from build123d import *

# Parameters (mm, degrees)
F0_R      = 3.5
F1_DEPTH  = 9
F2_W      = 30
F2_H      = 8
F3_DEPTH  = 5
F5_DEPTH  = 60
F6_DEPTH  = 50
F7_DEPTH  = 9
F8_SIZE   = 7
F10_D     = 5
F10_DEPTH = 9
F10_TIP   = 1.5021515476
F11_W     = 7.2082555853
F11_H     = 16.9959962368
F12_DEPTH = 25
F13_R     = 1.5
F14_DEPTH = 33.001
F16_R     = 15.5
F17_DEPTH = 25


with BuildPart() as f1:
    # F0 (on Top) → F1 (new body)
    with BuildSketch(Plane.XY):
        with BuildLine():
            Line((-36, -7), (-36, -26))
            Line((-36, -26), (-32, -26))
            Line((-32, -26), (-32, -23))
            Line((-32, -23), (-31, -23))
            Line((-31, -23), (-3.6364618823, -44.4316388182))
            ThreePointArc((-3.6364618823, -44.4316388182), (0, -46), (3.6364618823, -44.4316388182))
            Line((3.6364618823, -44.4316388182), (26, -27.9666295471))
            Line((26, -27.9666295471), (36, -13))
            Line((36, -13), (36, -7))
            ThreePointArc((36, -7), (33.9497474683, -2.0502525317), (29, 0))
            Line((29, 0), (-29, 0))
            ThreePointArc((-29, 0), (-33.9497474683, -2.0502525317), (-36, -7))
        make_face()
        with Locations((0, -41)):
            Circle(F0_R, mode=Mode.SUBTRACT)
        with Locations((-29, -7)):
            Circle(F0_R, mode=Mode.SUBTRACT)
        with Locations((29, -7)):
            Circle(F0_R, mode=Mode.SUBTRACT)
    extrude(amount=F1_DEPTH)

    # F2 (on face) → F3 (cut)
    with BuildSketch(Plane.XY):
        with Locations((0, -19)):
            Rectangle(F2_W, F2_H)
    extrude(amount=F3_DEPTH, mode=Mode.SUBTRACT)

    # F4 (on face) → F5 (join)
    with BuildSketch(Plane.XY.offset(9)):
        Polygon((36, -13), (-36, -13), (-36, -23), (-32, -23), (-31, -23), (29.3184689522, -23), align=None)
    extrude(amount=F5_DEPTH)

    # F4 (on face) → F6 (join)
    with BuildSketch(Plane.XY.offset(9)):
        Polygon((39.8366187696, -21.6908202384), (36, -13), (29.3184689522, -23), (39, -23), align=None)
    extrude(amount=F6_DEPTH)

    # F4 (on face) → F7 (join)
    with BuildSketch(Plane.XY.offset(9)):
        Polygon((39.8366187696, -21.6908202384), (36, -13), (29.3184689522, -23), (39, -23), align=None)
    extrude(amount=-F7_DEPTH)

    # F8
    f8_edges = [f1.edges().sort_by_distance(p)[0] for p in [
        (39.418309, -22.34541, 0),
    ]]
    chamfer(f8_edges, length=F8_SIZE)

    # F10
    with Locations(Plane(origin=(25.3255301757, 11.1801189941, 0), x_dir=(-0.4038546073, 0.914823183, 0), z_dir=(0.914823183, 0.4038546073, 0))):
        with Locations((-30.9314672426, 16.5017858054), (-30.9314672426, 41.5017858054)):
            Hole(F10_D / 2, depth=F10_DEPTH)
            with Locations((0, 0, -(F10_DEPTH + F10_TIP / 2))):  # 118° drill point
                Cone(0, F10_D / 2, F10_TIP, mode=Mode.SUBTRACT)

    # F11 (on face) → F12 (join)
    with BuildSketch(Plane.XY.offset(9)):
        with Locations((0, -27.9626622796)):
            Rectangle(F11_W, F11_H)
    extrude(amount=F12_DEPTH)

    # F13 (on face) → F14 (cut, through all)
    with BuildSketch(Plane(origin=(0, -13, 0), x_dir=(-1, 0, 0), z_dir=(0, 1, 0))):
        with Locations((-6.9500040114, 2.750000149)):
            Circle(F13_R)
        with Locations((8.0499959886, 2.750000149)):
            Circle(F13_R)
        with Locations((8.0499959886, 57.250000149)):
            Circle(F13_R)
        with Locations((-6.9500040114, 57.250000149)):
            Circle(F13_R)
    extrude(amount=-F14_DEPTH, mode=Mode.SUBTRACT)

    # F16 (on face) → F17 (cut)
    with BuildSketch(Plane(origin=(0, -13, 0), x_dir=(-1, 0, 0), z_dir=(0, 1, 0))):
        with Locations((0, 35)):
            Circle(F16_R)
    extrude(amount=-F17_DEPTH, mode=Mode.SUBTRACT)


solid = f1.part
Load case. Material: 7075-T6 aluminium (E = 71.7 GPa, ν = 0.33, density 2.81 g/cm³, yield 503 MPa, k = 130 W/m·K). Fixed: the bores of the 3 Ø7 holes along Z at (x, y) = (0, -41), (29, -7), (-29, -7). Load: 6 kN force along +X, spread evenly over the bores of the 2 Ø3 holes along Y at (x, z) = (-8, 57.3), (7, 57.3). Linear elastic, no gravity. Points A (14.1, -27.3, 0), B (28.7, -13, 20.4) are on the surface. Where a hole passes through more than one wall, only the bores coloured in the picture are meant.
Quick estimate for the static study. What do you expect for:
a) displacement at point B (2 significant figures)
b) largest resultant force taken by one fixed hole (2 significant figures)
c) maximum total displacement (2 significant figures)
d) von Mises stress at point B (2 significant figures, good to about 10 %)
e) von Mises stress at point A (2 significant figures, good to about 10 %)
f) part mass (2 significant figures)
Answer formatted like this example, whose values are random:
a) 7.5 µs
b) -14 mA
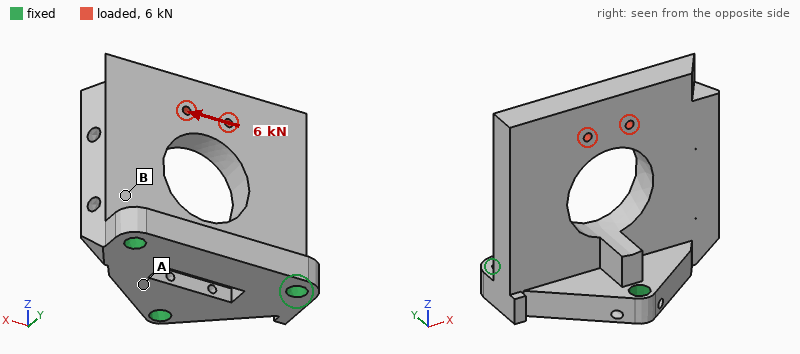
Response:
a) 0.036 mm
b) 5.7 kN
c) 0.13 mm
d) 52 MPa
e) 21 MPa
f) 160 g
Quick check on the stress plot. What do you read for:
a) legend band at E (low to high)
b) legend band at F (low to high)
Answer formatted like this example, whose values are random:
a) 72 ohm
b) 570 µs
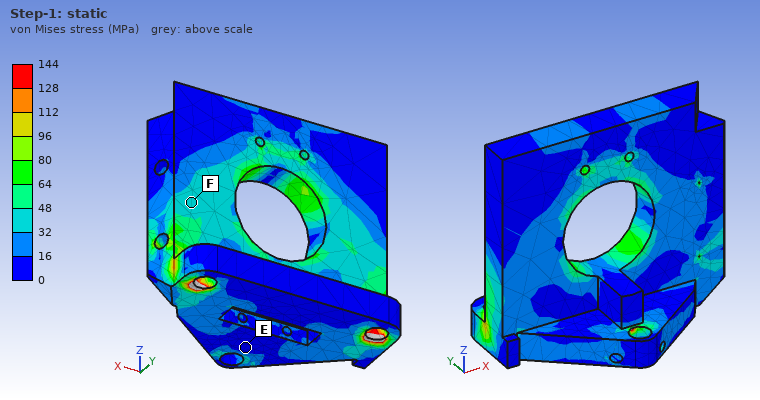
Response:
a) 0 to 16 MPa
b) 32 to 48 MPa
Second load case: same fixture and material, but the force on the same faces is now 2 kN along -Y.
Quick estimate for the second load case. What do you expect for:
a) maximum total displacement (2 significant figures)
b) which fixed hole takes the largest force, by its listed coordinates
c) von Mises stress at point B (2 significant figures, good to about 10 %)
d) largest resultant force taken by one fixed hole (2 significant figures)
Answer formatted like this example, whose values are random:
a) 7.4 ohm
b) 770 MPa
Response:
a) 0.46 mm
b) (0, -41)
c) 81 MPa
d) 3.4 kN
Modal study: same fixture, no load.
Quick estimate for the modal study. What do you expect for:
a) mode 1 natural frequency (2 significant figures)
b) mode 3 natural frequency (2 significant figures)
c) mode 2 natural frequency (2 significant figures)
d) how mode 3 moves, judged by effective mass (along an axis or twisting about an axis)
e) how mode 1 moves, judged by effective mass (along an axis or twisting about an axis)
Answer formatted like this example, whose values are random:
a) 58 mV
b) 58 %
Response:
a) 1700 Hz
b) 5300 Hz
c) 3400 Hz
d) along X
e) along Y
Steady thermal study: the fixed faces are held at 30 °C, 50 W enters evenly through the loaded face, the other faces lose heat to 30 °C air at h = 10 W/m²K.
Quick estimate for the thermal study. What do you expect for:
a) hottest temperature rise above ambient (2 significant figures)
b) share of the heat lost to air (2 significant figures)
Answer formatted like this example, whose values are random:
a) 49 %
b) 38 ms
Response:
a) 55 K
b) 6.7 %
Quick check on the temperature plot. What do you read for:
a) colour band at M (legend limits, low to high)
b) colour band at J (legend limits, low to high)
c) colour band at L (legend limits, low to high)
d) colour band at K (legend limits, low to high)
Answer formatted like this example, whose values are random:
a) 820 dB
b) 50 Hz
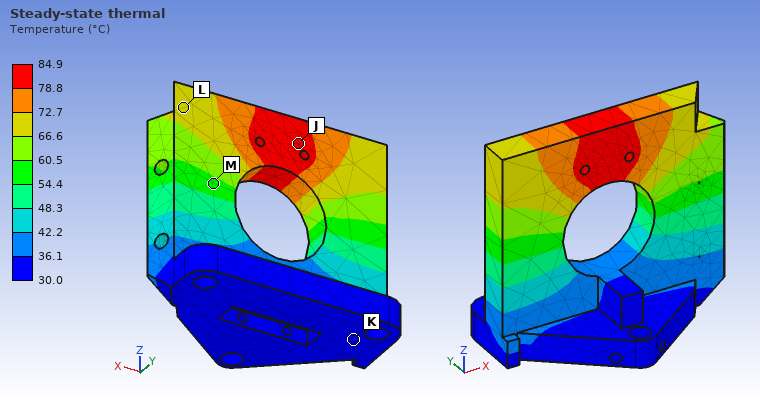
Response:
a) 54.4 to 60.5 °C
b) 78.8 to 84.9 °C
c) 66.6 to 72.7 °C
d) 30.0 to 36.1 °C
